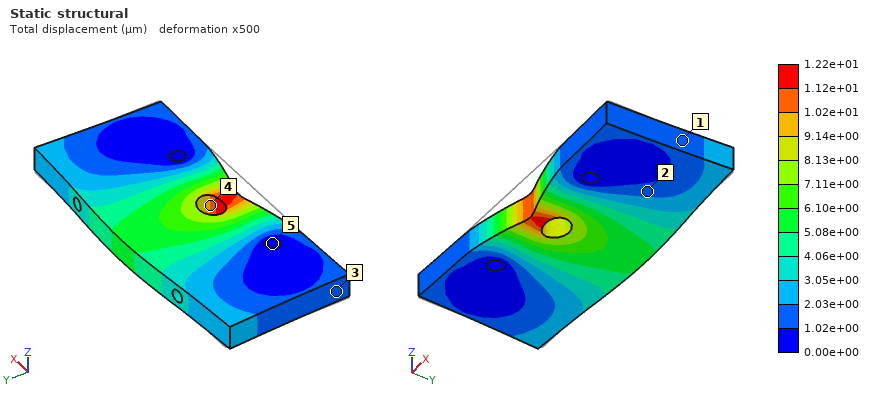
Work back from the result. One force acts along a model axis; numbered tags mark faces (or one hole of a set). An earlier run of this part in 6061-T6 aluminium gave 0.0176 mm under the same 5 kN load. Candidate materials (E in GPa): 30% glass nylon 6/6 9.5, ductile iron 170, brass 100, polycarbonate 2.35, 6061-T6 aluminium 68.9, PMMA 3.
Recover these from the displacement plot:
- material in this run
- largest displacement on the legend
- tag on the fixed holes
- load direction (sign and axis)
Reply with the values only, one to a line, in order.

brass
1.22e+01 µm
5
+Y
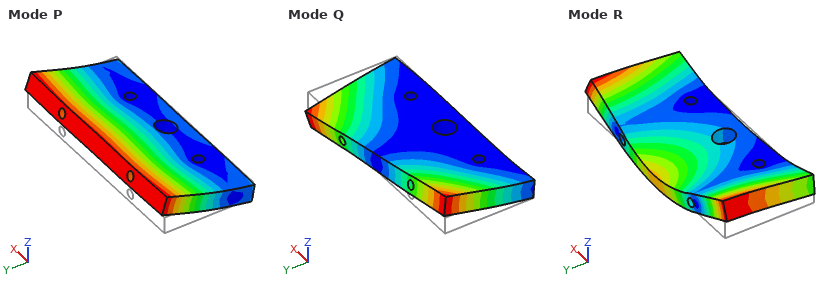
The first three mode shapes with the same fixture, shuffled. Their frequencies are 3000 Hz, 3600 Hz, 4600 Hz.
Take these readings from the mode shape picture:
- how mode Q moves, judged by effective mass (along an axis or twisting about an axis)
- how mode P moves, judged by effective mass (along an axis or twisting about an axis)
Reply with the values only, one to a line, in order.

twisting about Y
along Z
